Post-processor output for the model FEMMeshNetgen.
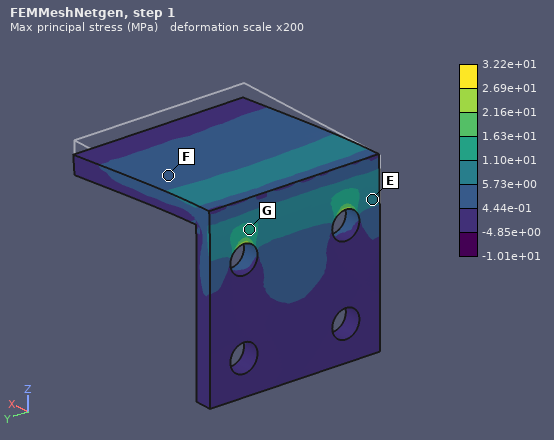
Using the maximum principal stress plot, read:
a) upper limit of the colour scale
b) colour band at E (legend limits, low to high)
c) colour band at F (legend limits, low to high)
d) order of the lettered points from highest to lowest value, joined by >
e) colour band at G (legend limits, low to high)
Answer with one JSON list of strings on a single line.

["3.22e+01 MPa", "5.73e+00 to 1.10e+01 MPa", "4.44e-01 to 5.73e+00 MPa", "G > E > F", "1.10e+01 to 1.63e+01 MPa"]
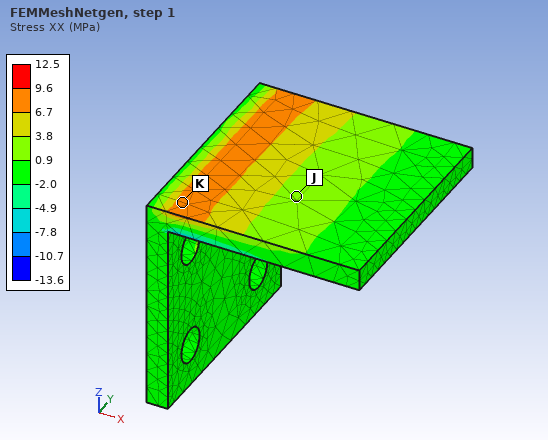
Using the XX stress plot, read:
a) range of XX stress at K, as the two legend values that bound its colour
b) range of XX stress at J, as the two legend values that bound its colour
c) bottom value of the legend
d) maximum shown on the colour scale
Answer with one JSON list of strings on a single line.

["6.7 to 9.6 MPa", "0.9 to 3.8 MPa", "-13.6 MPa", "12.5 MPa"]
